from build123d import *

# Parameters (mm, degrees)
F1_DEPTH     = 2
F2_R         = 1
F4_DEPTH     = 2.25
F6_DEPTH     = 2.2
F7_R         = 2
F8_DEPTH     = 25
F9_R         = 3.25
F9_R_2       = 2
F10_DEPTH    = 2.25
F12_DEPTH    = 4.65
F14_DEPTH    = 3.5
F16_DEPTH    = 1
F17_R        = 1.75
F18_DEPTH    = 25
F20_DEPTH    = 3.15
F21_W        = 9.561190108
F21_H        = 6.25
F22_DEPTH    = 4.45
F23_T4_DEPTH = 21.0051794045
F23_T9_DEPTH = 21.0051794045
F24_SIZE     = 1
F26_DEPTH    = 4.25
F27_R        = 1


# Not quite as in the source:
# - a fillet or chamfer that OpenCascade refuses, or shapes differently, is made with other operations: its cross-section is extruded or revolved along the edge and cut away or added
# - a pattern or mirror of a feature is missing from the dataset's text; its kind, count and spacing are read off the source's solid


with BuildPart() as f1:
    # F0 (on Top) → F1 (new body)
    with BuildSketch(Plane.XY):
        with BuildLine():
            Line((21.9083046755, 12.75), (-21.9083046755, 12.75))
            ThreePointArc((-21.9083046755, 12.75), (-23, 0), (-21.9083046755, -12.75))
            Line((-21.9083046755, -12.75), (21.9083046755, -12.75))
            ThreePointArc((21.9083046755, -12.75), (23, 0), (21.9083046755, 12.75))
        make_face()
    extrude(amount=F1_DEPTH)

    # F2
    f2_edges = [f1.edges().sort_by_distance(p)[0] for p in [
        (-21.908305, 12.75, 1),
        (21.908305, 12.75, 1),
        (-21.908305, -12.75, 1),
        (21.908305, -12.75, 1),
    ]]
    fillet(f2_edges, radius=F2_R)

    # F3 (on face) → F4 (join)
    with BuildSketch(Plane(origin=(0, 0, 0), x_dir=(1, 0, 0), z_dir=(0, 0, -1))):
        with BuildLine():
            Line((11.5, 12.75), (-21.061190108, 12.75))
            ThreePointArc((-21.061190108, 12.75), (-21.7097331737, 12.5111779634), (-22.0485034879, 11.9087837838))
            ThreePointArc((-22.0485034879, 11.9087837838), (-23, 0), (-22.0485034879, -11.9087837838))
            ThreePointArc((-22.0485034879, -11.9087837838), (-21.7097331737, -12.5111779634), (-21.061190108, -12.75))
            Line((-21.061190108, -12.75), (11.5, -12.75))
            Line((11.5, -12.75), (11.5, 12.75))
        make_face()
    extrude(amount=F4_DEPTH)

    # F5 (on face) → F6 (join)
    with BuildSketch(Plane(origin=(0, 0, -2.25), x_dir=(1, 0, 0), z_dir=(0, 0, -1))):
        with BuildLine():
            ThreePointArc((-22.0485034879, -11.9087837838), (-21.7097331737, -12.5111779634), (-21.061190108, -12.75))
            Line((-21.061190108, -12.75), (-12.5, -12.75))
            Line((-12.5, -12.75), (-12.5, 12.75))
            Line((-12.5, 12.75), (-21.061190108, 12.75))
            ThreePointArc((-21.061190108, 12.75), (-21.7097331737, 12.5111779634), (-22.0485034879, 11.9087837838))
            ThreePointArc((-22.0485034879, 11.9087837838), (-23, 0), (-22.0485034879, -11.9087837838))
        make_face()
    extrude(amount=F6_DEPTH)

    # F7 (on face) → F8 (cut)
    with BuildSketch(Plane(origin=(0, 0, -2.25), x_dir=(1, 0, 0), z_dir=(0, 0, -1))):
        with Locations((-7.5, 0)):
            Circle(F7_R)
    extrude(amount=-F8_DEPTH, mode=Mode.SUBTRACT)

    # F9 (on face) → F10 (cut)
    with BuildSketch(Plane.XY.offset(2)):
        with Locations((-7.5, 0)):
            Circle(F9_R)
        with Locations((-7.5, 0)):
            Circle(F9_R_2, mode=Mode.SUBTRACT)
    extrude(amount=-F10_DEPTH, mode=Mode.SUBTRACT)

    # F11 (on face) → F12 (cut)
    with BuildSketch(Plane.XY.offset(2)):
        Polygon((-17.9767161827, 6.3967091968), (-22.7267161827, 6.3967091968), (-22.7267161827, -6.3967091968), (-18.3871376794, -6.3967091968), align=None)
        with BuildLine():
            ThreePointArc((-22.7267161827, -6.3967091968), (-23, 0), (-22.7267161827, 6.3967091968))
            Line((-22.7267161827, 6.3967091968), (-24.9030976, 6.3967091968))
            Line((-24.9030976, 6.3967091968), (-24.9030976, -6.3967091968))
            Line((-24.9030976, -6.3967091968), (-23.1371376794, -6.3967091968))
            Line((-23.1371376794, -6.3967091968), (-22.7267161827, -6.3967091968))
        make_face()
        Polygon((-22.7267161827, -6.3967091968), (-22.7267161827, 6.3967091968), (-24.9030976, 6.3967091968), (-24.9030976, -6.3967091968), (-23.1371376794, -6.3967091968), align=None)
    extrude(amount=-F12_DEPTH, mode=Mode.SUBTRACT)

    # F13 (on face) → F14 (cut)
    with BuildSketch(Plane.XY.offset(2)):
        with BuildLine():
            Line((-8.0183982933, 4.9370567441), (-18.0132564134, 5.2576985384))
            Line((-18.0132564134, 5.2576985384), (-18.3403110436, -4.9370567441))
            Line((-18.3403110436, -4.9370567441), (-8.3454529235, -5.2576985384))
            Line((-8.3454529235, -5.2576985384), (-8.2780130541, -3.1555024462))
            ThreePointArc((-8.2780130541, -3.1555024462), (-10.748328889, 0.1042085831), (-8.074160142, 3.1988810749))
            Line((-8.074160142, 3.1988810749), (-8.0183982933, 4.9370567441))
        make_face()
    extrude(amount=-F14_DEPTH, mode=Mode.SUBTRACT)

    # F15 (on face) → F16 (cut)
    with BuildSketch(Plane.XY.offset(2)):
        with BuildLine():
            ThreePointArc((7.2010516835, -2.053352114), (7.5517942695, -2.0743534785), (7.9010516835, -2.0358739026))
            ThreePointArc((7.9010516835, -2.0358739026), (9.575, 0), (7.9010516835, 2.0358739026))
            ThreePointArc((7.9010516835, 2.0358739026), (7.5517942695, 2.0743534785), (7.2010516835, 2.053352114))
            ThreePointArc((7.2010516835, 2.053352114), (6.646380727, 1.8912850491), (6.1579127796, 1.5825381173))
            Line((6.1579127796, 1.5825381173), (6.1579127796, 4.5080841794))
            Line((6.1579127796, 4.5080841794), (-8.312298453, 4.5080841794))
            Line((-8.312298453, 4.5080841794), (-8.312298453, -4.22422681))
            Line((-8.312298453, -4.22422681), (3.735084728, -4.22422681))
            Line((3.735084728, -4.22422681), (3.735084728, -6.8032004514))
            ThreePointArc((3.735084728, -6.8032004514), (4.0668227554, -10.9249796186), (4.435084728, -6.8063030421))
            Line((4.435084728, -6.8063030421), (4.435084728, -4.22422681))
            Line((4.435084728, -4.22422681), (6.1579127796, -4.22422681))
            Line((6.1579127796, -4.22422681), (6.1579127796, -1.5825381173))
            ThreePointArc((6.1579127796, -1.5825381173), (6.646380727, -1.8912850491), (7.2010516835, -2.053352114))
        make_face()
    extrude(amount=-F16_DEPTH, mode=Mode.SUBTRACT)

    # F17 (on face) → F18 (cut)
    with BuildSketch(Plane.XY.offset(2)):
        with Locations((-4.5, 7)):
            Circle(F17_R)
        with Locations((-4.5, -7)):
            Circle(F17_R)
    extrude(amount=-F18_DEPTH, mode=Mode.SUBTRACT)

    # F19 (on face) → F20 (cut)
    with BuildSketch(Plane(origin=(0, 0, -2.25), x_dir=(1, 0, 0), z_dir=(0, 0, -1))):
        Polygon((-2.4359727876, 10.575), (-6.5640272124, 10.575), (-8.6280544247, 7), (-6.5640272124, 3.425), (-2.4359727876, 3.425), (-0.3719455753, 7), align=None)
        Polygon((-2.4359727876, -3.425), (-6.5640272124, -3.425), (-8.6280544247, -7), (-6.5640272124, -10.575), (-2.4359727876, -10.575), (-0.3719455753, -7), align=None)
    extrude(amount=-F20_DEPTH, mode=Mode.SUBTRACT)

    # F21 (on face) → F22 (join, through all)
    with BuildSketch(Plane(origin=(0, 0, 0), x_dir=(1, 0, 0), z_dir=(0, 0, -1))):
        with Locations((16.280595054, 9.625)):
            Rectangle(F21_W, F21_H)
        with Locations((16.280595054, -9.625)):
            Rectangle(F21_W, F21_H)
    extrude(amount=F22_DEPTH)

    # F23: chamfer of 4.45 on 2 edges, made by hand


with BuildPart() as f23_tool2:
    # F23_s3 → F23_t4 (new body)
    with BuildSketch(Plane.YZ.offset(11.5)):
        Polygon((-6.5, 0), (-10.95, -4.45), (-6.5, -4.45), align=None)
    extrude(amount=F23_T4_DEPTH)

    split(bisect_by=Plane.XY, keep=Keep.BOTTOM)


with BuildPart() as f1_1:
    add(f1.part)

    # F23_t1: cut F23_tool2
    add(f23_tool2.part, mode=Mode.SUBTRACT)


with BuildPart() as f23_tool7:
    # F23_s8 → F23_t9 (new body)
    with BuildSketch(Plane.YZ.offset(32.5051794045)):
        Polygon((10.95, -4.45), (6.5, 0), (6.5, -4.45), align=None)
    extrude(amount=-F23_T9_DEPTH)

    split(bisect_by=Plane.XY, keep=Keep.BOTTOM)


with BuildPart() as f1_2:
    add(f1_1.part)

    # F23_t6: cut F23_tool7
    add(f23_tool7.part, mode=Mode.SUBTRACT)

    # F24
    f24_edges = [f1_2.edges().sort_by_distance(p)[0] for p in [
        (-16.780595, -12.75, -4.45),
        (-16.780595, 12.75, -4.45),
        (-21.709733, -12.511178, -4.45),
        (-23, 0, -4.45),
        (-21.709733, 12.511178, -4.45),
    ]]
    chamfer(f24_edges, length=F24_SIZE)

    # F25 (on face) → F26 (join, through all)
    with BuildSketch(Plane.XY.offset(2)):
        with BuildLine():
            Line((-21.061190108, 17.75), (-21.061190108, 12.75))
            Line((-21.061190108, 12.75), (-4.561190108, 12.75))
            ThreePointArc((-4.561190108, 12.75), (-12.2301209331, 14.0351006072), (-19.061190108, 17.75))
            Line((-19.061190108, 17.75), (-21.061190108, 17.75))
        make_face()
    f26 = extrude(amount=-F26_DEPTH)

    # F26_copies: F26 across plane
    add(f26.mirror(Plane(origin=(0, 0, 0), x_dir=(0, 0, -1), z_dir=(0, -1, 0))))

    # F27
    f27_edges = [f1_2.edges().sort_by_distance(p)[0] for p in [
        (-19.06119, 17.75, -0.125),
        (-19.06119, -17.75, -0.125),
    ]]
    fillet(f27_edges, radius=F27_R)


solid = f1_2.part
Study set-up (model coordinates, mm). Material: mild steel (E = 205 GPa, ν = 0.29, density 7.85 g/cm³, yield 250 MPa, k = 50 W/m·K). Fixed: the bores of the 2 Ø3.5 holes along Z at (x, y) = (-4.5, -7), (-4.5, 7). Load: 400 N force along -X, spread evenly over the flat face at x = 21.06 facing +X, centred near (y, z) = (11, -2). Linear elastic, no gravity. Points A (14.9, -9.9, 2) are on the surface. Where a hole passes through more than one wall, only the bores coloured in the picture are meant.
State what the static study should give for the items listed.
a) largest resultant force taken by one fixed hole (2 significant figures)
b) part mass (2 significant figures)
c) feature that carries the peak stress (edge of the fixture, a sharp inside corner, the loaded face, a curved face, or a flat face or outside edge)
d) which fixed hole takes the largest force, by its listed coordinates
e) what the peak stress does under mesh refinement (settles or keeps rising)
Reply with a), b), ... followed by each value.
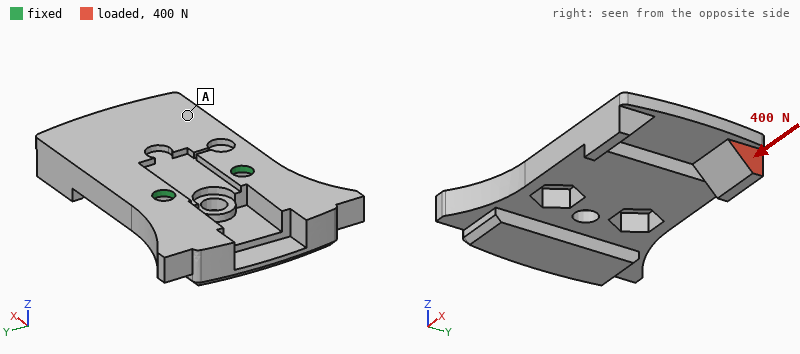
a) 450 N
b) 34 g
c) edge of the fixture
d) (-4.5, 7)
e) keeps rising
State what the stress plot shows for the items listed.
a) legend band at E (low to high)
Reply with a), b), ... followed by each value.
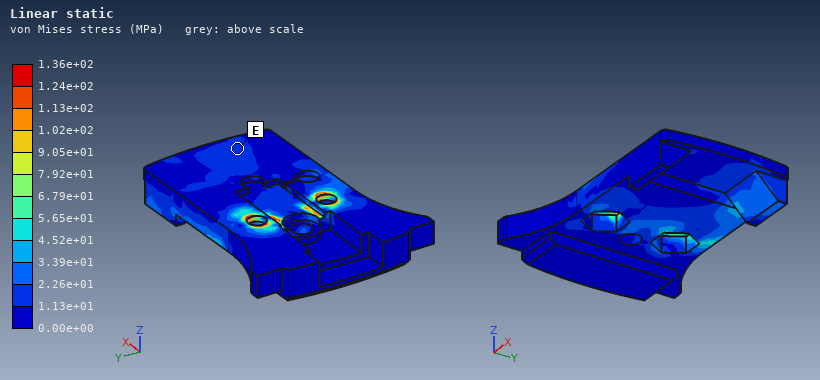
a) 1.13e+01 to 2.26e+01 MPa
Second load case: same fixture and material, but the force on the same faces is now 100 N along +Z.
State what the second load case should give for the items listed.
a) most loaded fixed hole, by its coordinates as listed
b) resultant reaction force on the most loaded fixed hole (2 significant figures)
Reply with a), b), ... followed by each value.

a) (-4.5, 7)
b) 120 N
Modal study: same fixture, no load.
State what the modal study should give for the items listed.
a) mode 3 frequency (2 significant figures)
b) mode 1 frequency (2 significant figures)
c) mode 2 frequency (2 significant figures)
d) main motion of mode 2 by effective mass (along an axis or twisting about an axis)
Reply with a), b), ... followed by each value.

a) 6600 Hz
b) 2200 Hz
c) 5600 Hz
d) along Z
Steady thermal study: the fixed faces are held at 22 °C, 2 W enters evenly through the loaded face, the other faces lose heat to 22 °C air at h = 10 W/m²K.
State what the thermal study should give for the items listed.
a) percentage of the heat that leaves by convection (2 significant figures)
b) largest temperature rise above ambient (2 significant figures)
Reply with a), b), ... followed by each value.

a) 9.5 %
b) 24 K
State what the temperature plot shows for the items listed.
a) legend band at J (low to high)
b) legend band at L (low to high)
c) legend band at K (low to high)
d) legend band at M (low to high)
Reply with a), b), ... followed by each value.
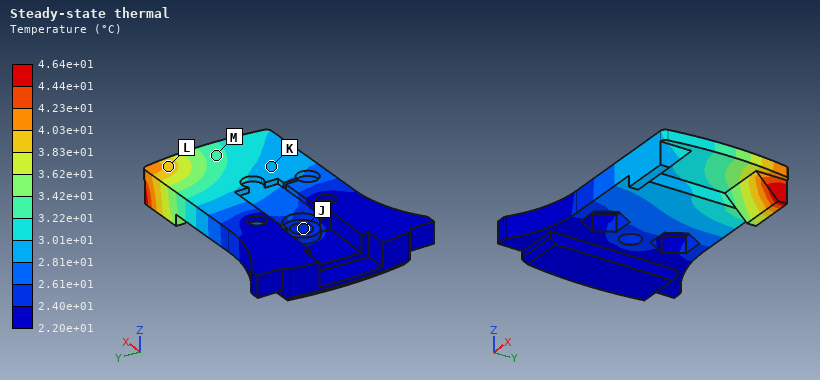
a) 2.40e+01 to 2.61e+01 °C
b) 3.83e+01 to 4.03e+01 °C
c) 2.81e+01 to 3.01e+01 °C
d) 3.22e+01 to 3.42e+01 °C
